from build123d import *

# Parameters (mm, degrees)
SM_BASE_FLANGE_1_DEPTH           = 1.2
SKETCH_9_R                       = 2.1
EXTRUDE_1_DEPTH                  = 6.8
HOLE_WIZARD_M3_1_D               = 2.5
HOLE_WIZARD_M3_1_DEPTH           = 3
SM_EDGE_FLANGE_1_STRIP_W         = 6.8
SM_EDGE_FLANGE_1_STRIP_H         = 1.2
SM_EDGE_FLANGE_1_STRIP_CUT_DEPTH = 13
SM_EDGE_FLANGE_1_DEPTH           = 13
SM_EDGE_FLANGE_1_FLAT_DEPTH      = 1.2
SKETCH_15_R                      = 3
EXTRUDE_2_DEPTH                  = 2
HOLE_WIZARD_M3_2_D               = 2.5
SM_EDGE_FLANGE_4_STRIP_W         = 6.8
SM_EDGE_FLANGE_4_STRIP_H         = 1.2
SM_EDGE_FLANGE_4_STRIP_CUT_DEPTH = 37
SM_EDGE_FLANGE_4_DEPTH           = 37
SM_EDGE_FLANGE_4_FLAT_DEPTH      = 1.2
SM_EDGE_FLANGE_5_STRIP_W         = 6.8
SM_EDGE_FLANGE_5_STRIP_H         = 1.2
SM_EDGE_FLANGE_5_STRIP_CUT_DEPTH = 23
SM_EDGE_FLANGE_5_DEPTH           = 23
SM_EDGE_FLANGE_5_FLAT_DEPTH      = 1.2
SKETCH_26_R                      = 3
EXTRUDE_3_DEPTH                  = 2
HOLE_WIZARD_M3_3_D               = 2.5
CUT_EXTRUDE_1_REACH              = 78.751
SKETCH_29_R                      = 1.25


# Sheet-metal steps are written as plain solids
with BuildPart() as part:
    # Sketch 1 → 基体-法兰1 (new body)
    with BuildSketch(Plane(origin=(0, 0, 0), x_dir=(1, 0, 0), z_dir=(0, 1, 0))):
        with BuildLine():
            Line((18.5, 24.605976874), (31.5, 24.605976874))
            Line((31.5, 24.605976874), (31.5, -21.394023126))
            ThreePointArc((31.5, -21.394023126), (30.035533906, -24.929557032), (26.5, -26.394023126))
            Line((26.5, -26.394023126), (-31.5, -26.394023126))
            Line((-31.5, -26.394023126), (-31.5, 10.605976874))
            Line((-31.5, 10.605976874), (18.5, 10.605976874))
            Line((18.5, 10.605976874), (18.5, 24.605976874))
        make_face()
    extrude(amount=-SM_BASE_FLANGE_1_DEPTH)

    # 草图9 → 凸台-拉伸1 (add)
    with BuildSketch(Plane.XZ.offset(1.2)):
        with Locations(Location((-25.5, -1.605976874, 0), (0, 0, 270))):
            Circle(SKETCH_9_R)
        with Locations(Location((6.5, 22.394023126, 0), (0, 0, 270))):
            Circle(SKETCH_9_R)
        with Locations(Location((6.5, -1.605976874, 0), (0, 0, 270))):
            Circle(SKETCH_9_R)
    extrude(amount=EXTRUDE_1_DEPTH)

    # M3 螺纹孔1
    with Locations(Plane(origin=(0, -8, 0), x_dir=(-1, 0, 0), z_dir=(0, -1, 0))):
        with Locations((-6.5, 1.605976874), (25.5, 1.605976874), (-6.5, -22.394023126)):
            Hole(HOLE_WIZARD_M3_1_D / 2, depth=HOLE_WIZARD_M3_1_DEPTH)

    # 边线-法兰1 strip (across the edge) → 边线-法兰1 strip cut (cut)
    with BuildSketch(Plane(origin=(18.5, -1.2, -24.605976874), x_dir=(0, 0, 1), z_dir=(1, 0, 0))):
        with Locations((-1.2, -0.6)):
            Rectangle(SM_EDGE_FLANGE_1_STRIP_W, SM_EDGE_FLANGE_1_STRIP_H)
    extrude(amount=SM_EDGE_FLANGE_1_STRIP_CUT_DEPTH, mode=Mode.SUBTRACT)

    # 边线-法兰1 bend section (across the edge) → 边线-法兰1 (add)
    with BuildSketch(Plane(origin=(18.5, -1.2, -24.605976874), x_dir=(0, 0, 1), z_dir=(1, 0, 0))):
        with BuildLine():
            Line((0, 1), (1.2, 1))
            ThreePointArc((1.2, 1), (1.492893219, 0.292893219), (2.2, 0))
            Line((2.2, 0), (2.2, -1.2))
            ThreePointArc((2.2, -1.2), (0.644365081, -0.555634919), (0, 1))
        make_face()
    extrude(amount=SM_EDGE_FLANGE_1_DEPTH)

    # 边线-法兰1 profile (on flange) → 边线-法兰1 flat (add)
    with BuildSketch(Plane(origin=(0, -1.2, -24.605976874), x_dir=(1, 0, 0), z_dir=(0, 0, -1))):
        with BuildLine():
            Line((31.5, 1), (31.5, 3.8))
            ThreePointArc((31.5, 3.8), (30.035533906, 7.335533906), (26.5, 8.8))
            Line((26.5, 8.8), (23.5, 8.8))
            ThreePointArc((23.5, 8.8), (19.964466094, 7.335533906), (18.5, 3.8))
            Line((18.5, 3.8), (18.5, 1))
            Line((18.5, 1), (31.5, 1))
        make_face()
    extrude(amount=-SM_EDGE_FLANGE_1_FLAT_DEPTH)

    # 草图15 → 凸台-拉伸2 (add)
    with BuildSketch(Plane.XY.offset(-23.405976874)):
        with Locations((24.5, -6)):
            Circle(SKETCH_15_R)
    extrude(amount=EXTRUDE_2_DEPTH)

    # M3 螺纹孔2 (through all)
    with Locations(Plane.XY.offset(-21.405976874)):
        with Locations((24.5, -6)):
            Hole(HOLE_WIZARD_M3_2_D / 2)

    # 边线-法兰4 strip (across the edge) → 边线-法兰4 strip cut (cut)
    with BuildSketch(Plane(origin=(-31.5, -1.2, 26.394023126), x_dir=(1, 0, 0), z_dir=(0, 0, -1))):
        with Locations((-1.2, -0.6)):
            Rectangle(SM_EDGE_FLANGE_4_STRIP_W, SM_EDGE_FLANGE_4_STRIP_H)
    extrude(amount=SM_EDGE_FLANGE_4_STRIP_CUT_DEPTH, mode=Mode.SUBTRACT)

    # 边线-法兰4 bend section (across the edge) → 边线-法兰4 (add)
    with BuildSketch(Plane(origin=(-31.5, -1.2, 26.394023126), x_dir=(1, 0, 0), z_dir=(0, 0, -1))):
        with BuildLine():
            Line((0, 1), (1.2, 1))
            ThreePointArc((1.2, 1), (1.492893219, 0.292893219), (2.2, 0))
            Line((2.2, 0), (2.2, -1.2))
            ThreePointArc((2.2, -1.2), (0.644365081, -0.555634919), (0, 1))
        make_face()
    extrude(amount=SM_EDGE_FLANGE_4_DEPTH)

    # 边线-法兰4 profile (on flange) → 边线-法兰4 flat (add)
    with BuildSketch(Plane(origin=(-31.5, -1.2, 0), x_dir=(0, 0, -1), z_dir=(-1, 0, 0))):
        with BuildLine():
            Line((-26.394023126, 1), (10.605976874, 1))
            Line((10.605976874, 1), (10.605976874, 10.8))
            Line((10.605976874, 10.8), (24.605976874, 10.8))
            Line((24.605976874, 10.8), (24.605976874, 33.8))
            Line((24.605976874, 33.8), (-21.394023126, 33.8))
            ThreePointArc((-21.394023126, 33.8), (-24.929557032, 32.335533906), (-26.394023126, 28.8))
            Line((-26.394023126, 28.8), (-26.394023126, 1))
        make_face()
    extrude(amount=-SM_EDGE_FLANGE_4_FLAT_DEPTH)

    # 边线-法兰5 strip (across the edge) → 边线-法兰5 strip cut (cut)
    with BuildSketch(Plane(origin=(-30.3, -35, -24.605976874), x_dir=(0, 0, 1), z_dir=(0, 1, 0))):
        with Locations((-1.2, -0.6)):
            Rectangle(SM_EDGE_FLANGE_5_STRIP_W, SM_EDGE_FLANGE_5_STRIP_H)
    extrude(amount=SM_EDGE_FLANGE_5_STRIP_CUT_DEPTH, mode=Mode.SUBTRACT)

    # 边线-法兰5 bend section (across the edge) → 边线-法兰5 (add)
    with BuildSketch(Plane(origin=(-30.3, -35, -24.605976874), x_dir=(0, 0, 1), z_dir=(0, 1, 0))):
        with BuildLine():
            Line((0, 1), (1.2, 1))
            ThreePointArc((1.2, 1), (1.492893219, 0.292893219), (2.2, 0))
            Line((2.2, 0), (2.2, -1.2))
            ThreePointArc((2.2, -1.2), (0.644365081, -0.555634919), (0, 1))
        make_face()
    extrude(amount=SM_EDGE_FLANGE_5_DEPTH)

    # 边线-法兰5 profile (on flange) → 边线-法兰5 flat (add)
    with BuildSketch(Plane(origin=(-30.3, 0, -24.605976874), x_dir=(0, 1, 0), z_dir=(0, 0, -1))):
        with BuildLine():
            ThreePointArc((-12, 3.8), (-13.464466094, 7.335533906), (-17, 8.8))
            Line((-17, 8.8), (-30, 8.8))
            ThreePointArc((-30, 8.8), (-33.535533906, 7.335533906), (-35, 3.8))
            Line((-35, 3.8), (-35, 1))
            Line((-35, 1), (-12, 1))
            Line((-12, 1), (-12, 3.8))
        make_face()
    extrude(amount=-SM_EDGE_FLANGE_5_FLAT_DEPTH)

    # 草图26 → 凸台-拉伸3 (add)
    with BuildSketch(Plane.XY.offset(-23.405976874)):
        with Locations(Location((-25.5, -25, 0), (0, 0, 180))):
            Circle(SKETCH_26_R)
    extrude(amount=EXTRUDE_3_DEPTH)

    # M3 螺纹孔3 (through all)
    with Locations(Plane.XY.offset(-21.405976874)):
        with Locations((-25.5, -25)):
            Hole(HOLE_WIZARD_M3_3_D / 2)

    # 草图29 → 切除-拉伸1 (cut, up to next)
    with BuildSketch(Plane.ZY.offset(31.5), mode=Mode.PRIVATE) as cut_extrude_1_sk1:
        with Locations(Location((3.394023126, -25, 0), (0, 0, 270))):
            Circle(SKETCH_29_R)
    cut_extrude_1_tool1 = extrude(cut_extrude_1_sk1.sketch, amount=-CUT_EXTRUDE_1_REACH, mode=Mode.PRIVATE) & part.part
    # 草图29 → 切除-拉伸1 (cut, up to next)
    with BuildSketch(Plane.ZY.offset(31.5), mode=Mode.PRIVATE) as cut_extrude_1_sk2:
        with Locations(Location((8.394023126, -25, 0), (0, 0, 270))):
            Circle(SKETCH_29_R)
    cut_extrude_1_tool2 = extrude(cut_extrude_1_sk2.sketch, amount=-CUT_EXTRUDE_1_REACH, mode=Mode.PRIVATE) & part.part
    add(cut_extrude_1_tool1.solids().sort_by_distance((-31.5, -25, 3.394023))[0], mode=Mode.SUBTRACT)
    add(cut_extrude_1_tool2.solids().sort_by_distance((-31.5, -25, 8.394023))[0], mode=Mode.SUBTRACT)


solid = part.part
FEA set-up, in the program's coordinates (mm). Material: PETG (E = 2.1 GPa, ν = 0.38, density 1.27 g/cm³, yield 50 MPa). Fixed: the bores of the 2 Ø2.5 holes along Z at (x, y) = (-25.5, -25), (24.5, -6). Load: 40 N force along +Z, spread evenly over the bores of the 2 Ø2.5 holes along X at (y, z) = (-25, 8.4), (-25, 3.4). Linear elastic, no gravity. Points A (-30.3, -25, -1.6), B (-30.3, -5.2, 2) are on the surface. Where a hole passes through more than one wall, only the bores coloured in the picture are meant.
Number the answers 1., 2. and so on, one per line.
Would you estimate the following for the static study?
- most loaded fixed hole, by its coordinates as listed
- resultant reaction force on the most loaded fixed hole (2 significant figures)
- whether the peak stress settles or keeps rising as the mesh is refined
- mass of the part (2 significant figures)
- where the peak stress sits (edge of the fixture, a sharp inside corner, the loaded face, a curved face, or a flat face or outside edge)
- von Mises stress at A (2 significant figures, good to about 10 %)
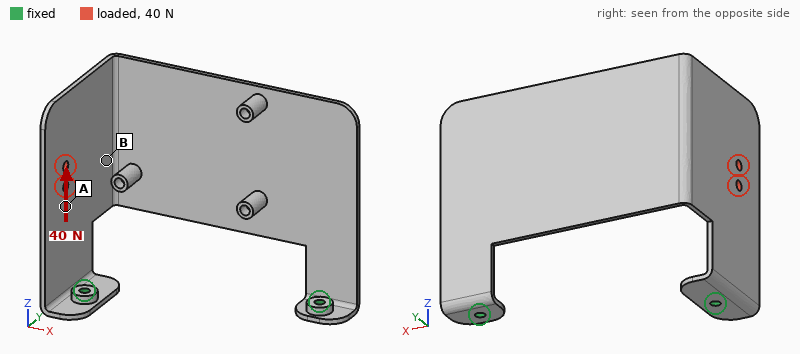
1. (-25.5, -25)
2. 40 N
3. keeps rising
4. 7.0 g
5. edge of the fixture
6. 3.0 MPa
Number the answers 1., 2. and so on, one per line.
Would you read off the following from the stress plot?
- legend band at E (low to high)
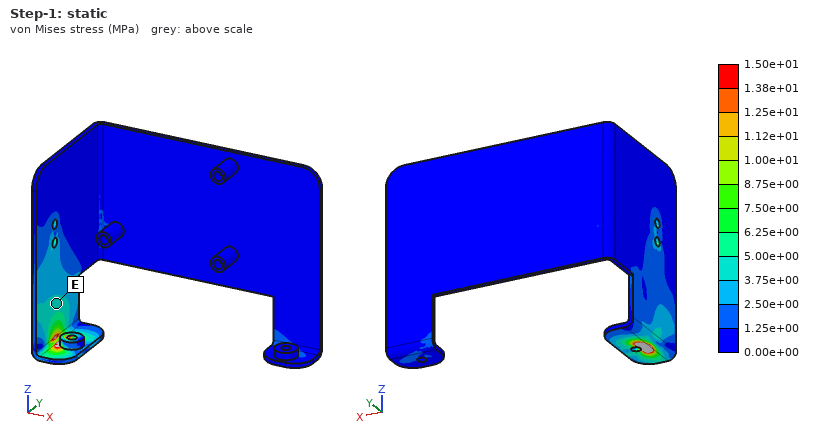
1. 3.75e+00 to 5.00e+00 MPa
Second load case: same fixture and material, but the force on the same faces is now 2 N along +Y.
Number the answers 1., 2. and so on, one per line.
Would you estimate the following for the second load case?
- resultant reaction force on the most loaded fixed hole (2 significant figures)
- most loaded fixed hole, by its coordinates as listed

1. 2.0 N
2. (-25.5, -25)
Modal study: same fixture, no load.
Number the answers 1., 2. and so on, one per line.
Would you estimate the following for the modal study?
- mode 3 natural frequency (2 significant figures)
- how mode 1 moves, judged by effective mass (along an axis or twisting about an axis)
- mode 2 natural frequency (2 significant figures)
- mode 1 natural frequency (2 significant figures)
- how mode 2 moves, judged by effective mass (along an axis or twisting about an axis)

1. 240 Hz
2. along Y
3. 150 Hz
4. 96 Hz
5. along X
